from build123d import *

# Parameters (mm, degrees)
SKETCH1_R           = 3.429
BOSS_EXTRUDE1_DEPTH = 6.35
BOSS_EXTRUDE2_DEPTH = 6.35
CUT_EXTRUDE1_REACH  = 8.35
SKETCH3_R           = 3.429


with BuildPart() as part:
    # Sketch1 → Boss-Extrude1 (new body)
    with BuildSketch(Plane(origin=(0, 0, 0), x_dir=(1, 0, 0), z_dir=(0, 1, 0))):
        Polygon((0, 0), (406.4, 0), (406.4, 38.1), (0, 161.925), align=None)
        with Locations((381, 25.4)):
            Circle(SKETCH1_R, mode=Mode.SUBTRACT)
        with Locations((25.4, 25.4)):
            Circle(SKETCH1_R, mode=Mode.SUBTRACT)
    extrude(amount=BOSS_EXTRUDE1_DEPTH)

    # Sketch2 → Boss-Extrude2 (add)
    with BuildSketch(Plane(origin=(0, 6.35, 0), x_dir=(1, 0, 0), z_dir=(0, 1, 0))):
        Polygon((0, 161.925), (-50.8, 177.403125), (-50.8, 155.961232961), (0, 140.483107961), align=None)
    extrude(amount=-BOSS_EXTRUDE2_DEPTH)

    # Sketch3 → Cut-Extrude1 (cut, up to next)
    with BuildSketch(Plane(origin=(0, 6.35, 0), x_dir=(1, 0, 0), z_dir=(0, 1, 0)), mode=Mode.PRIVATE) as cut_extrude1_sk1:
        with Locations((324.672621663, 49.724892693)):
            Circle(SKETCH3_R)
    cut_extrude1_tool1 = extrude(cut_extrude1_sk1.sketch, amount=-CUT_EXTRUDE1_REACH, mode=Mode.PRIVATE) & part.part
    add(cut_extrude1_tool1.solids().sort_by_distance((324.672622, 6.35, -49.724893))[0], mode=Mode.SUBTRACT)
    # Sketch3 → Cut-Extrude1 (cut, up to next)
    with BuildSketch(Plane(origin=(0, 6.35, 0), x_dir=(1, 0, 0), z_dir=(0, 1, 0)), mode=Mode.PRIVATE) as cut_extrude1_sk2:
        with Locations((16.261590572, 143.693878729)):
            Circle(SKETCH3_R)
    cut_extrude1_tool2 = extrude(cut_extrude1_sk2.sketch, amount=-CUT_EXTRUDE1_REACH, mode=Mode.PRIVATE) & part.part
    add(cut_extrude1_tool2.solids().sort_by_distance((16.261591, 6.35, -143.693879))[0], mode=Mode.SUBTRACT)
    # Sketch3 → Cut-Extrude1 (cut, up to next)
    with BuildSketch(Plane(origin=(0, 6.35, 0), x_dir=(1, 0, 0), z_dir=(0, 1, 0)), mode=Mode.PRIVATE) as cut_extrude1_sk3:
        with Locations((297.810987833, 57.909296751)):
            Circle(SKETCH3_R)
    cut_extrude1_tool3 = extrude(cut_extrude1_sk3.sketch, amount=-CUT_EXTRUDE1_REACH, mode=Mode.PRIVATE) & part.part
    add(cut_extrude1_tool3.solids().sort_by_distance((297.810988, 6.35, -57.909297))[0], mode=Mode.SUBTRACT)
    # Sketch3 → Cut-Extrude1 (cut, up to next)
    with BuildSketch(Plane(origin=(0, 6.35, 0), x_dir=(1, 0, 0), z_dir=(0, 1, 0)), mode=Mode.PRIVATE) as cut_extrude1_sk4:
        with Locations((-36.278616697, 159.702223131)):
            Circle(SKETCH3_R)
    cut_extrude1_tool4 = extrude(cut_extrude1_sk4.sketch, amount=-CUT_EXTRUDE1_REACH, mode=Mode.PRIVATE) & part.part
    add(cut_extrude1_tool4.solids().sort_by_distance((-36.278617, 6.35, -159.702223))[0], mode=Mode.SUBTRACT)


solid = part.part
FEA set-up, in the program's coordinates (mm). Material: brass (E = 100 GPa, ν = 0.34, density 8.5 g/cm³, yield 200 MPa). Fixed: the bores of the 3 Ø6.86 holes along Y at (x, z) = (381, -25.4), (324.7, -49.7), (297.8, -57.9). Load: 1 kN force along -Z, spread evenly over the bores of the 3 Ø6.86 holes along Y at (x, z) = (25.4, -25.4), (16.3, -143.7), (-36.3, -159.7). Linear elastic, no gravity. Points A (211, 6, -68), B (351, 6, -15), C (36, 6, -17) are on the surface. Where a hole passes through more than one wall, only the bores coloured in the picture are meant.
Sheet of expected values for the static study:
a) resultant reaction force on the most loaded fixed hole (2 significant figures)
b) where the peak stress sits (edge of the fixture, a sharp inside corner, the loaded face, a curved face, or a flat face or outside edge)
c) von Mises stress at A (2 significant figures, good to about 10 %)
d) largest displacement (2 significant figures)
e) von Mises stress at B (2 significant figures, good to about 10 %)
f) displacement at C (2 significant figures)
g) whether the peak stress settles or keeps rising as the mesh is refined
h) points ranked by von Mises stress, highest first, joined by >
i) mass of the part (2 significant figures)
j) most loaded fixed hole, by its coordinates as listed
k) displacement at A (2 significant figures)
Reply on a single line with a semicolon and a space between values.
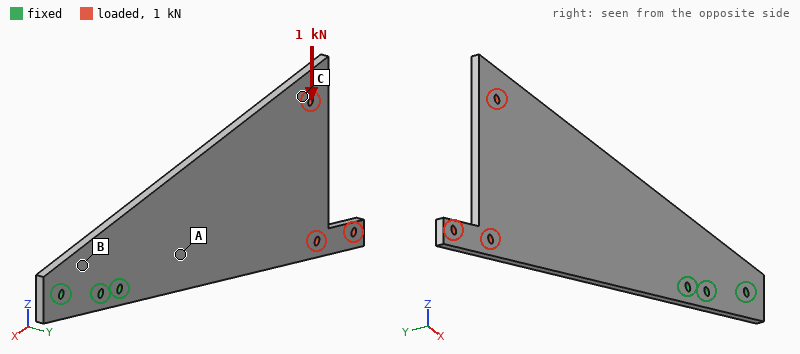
6.4 kN; edge of the fixture; 10 MPa; 0.60 mm; 19 MPa; 0.36 mm; keeps rising; B > A > C; 2.2 kg; (297.8, -57.9); 0.097 mm
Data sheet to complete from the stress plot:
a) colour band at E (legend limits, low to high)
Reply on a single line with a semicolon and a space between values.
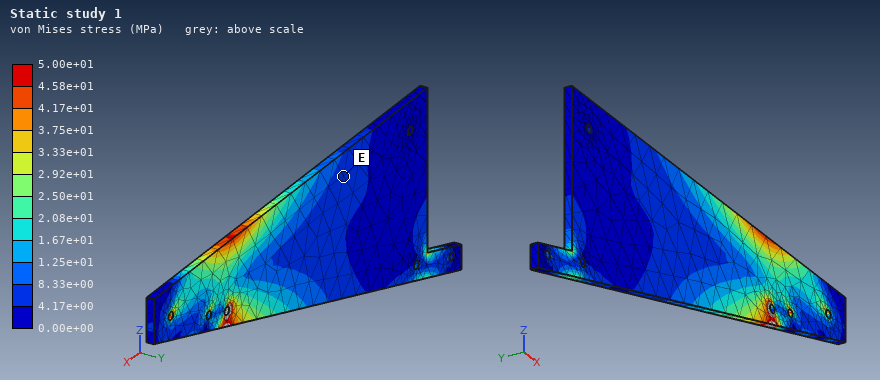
4.17e+00 to 8.33e+00 MPa
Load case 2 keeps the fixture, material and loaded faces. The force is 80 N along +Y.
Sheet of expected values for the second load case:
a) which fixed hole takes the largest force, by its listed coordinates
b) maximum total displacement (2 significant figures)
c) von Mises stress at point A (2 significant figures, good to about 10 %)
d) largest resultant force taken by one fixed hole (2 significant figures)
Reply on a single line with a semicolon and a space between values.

(297.8, -57.9); 5.3 mm; 26 MPa; 460 N
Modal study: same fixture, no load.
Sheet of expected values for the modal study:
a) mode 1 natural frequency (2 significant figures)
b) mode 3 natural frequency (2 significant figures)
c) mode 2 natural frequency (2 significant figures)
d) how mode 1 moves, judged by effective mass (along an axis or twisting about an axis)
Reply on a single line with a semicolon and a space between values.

28 Hz; 210 Hz; 120 Hz; along Y
